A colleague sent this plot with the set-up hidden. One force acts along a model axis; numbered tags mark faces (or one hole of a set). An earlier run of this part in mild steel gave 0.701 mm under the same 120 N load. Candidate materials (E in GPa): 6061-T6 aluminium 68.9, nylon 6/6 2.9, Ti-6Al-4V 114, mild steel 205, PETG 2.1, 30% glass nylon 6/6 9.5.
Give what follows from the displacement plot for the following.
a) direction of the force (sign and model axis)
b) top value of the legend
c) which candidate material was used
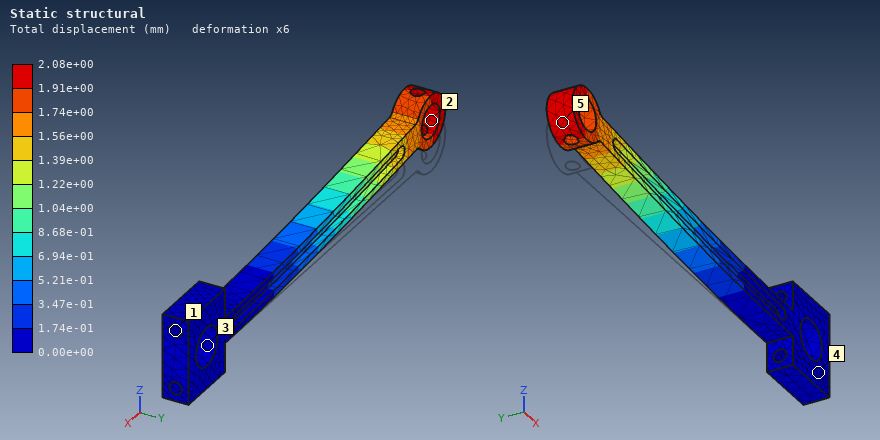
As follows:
+Z
2.08e+00 mm
6061-T6 aluminium
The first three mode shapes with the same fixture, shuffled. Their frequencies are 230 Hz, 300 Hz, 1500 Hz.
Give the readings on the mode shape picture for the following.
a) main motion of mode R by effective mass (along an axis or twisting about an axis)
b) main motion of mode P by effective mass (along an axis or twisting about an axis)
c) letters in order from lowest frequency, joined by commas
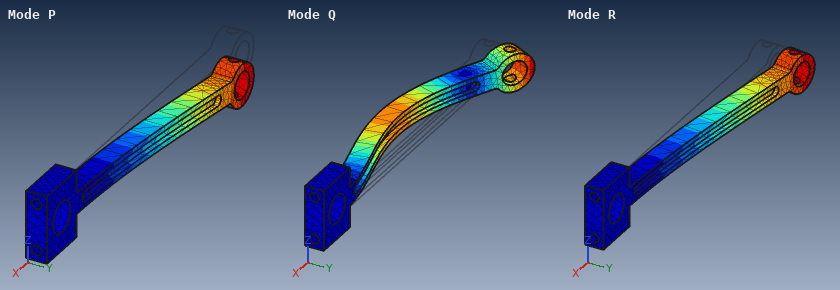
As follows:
along Y
along Z
R, P, Q
